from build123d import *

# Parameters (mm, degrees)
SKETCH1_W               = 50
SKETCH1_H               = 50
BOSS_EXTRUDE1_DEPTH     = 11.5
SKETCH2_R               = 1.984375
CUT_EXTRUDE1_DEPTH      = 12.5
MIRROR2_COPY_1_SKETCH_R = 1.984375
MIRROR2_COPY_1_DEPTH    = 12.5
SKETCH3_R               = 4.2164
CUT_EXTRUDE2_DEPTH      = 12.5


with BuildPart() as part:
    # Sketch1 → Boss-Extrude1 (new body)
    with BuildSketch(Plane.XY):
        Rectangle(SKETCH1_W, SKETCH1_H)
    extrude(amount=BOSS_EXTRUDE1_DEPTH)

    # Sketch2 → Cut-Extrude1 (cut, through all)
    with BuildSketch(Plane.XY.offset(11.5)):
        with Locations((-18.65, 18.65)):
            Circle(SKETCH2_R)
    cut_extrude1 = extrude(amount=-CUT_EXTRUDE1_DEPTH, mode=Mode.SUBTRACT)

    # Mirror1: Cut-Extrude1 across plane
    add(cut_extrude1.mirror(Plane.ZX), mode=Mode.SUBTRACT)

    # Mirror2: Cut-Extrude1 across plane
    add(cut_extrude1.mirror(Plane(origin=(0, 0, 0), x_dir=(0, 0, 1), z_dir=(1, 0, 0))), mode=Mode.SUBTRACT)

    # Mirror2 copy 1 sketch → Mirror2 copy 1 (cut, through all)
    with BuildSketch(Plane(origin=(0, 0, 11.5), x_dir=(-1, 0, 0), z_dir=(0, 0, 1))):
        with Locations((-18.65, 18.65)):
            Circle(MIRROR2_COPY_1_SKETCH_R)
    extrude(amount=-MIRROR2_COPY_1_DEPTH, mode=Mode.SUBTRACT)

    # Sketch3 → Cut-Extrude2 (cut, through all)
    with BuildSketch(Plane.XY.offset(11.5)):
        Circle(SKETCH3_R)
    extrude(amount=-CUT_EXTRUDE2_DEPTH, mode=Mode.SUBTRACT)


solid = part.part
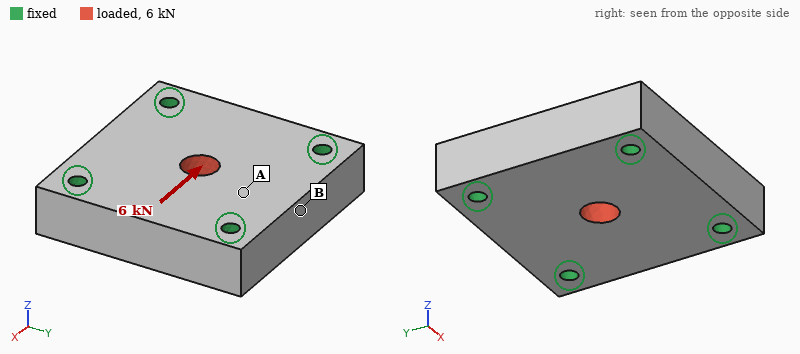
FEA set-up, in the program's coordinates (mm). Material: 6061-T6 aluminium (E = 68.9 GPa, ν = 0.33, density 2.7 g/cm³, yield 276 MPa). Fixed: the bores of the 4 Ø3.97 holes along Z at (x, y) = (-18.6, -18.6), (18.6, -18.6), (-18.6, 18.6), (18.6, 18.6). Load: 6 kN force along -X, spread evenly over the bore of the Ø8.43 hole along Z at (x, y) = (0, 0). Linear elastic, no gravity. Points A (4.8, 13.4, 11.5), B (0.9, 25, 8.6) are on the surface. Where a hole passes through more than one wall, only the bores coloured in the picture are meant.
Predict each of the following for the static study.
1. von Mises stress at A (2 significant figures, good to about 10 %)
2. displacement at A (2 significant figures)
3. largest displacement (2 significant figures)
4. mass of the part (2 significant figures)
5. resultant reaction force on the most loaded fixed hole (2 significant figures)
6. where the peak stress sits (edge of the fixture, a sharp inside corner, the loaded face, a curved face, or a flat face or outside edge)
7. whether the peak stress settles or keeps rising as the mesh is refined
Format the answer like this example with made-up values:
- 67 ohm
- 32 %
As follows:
- 8.3 MPa
- 1.9 µm
- 5.6 µm
- 74 g
- 1.7 kN
- edge of the fixture
- keeps rising
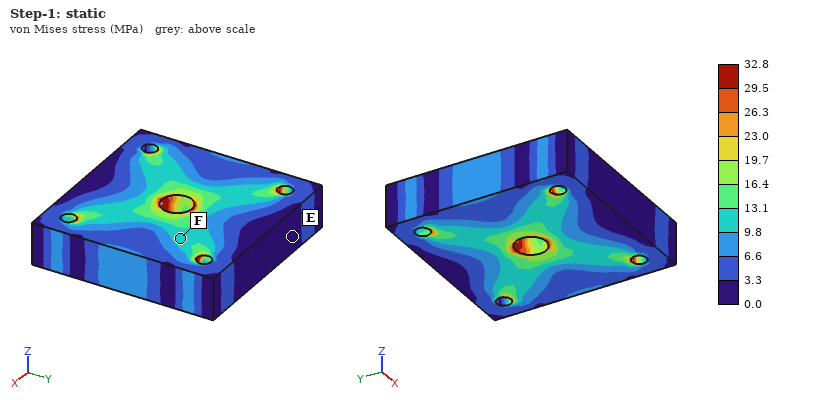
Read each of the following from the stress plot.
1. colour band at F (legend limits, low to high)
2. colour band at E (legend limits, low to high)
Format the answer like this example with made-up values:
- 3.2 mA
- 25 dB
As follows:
- 9.8 to 13.1 MPa
- 0.0 to 3.3 MPa
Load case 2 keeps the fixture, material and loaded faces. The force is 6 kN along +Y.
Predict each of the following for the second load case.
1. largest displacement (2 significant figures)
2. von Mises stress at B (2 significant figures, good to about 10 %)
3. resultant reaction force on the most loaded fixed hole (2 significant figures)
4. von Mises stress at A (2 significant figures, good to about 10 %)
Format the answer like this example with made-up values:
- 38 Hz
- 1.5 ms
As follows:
- 5.6 µm
- 9.0 MPa
- 1.7 kN
- 9.0 MPa
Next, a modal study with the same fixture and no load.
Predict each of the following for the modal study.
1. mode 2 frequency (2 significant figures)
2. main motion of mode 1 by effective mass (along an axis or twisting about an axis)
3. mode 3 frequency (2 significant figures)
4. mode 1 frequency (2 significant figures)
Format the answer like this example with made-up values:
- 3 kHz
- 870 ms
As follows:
- 30 kHz
- along Z
- 30 kHz
- 21 kHz
